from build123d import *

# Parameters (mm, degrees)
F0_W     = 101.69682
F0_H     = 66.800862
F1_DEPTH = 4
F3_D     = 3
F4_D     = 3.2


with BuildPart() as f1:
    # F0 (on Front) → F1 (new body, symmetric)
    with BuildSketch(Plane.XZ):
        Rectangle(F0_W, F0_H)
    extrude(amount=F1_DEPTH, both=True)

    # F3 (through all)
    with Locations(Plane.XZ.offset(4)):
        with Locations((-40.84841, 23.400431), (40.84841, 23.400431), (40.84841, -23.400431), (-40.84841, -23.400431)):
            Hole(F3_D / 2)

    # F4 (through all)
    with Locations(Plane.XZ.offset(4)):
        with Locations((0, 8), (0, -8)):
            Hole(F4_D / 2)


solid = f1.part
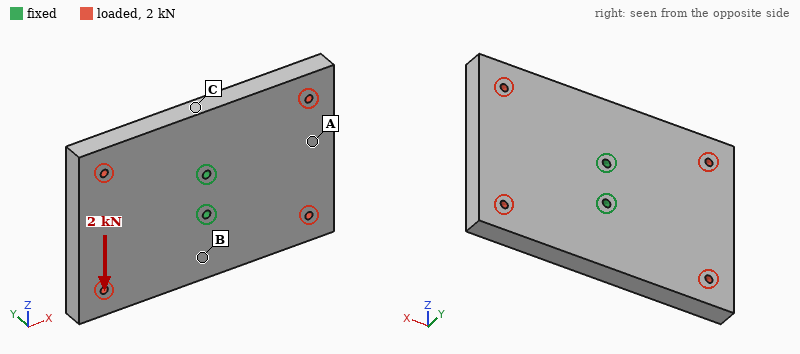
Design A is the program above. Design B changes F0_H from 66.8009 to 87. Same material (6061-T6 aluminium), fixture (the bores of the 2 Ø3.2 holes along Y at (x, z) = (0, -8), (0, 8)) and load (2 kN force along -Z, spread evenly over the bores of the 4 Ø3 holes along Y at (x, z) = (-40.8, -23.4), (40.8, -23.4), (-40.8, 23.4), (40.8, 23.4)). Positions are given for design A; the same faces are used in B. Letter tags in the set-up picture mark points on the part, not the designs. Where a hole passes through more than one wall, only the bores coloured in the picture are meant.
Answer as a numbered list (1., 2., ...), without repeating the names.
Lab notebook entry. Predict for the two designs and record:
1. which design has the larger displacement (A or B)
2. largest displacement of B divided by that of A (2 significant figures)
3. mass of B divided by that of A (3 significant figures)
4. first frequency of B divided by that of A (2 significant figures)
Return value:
1. A
2. 0.71
3. 1.30
4. 0.87
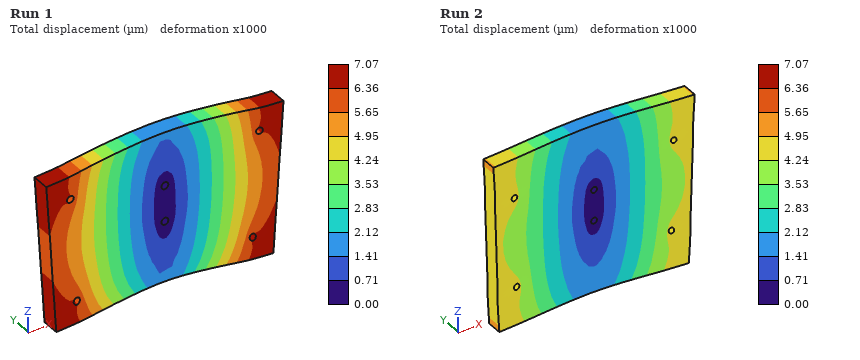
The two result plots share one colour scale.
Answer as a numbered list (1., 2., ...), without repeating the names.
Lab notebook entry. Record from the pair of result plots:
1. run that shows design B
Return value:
1. Run 2
